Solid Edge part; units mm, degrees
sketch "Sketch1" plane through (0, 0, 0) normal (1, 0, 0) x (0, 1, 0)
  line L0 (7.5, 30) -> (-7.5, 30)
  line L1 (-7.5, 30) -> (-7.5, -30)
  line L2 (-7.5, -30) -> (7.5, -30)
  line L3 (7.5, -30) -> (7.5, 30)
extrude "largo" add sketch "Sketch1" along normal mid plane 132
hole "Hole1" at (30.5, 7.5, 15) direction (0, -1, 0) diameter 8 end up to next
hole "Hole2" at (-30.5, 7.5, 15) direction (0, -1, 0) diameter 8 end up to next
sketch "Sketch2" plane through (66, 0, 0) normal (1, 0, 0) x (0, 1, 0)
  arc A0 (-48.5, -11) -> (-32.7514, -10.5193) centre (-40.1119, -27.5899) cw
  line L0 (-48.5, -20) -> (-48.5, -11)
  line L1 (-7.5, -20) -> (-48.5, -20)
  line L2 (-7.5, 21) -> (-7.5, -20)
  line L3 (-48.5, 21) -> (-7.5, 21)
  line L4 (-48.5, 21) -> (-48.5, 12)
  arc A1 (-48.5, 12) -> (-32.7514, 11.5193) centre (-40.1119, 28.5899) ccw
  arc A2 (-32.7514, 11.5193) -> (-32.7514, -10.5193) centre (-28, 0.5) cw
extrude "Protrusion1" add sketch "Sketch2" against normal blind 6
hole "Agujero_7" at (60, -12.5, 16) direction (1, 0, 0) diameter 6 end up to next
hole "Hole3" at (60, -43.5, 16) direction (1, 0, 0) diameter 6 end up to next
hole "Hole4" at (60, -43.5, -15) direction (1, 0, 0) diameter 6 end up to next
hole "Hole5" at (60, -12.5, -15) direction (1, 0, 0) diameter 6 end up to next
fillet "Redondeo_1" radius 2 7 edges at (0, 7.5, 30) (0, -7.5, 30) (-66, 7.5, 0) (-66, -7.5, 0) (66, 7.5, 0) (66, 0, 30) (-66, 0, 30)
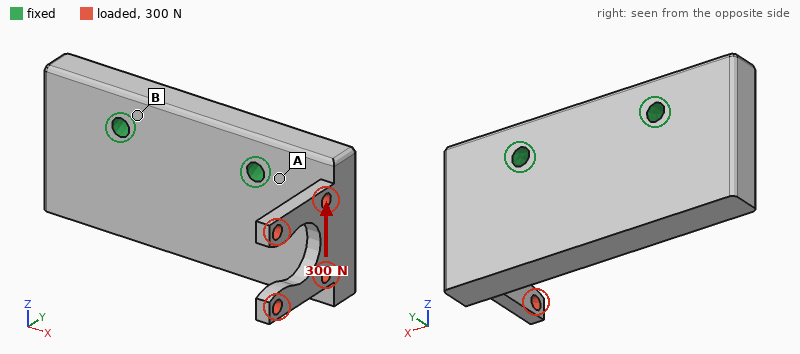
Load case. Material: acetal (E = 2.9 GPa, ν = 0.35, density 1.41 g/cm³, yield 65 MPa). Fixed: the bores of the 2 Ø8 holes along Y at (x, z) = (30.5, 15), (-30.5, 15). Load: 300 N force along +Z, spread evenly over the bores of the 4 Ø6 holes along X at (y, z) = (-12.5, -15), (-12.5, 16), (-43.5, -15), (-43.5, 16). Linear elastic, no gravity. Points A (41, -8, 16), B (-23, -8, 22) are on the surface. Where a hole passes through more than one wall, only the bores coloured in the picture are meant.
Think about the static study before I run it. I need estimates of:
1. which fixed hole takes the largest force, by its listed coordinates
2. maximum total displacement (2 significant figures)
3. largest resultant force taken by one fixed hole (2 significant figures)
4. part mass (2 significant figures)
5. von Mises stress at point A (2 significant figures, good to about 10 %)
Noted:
(30.5, 15)
1.1 mm
440 N
170 g
4.6 MPa
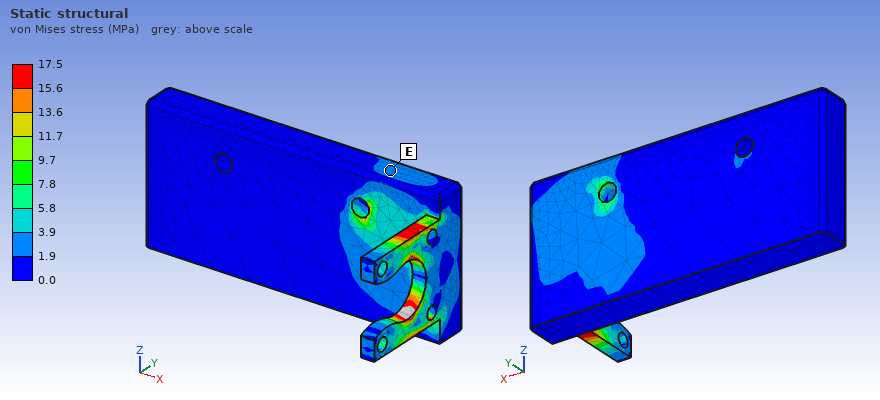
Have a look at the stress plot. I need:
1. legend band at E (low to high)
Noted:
1.9 to 3.9 MPa
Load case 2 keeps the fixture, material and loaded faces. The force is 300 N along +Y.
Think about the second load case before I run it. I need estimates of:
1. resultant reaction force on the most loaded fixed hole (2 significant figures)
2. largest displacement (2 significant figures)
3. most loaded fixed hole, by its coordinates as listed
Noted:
360 N
0.34 mm
(30.5, 15)
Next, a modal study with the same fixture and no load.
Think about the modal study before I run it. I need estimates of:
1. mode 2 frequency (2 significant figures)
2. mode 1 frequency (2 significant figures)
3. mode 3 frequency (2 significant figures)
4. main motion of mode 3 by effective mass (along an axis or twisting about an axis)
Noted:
870 Hz
810 Hz
1100 Hz
along Y
